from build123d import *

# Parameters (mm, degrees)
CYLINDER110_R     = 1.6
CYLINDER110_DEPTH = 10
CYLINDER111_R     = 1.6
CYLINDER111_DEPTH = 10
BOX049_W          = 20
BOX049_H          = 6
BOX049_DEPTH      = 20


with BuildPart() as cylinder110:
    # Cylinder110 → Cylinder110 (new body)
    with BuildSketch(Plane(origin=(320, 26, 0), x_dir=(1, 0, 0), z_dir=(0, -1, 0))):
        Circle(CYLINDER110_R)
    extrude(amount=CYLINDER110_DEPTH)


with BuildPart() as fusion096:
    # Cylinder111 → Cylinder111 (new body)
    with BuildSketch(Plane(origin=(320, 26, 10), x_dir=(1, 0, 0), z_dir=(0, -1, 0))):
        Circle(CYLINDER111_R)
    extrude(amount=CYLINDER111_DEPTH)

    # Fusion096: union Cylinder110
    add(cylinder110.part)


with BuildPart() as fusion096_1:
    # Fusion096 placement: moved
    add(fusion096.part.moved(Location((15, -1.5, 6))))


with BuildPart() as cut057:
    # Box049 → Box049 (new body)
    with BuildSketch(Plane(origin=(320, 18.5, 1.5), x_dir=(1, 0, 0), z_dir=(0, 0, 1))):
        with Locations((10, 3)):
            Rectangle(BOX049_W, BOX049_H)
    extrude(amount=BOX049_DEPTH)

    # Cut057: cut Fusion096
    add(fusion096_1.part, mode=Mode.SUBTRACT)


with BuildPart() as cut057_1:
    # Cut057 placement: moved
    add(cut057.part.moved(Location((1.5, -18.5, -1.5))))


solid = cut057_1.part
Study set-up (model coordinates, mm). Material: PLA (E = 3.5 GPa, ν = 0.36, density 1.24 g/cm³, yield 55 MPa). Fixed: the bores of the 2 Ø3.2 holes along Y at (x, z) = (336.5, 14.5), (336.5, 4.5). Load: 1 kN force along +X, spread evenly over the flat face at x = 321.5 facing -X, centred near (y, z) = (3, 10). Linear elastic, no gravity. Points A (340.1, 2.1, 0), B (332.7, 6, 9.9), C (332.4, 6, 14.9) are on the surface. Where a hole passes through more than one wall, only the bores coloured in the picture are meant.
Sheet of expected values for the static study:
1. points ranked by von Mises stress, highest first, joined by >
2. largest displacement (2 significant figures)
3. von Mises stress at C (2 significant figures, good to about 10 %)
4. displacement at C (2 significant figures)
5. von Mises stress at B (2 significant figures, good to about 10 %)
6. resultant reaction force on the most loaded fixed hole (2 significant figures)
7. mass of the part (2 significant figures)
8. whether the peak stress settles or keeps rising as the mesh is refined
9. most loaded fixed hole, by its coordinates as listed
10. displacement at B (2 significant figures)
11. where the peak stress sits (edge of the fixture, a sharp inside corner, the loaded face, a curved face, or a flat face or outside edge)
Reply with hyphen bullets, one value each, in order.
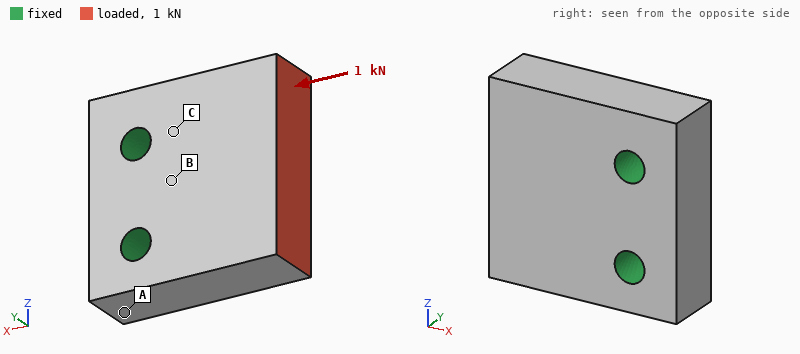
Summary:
- C > B > A
- 42 µm
- 11 MPa
- 11 µm
- 5.6 MPa
- 540 N
- 2.9 g
- keeps rising
- (336.5, 14.5)
- 11 µm
- edge of the fixture
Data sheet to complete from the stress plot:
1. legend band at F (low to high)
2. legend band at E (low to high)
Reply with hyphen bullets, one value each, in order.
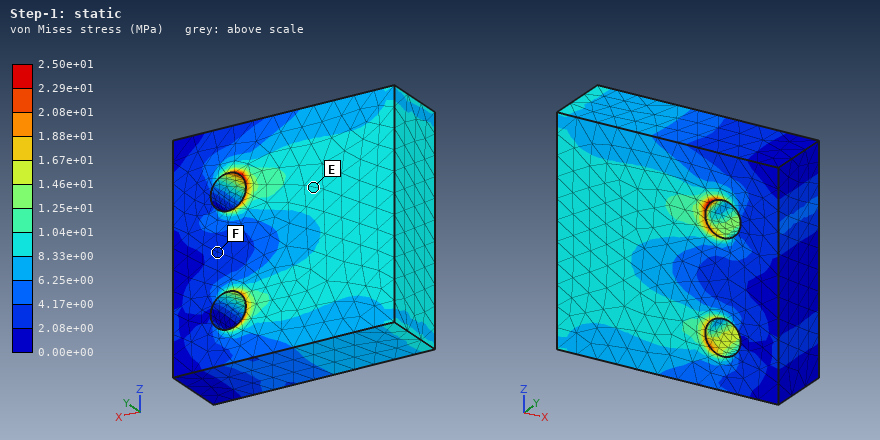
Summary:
- 2.08e+00 to 4.17e+00 MPa
- 8.33e+00 to 1.04e+01 MPa
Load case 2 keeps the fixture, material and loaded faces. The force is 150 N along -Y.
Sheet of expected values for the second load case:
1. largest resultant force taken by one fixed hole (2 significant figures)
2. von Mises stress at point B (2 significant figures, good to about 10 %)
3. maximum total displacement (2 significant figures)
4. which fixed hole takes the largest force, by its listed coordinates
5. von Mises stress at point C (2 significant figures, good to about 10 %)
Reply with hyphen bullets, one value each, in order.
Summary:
- 80 N
- 10 MPa
- 0.15 mm
- (336.5, 14.5)
- 15 MPa
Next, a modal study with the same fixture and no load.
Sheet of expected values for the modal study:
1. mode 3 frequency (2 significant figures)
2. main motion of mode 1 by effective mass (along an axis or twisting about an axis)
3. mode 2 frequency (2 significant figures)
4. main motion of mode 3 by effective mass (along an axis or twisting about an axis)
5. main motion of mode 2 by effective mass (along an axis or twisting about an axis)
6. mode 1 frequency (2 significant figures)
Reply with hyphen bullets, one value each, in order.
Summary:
- 12 kHz
- along Y
- 11 kHz
- along Z
- twisting about X
- 6800 Hz
